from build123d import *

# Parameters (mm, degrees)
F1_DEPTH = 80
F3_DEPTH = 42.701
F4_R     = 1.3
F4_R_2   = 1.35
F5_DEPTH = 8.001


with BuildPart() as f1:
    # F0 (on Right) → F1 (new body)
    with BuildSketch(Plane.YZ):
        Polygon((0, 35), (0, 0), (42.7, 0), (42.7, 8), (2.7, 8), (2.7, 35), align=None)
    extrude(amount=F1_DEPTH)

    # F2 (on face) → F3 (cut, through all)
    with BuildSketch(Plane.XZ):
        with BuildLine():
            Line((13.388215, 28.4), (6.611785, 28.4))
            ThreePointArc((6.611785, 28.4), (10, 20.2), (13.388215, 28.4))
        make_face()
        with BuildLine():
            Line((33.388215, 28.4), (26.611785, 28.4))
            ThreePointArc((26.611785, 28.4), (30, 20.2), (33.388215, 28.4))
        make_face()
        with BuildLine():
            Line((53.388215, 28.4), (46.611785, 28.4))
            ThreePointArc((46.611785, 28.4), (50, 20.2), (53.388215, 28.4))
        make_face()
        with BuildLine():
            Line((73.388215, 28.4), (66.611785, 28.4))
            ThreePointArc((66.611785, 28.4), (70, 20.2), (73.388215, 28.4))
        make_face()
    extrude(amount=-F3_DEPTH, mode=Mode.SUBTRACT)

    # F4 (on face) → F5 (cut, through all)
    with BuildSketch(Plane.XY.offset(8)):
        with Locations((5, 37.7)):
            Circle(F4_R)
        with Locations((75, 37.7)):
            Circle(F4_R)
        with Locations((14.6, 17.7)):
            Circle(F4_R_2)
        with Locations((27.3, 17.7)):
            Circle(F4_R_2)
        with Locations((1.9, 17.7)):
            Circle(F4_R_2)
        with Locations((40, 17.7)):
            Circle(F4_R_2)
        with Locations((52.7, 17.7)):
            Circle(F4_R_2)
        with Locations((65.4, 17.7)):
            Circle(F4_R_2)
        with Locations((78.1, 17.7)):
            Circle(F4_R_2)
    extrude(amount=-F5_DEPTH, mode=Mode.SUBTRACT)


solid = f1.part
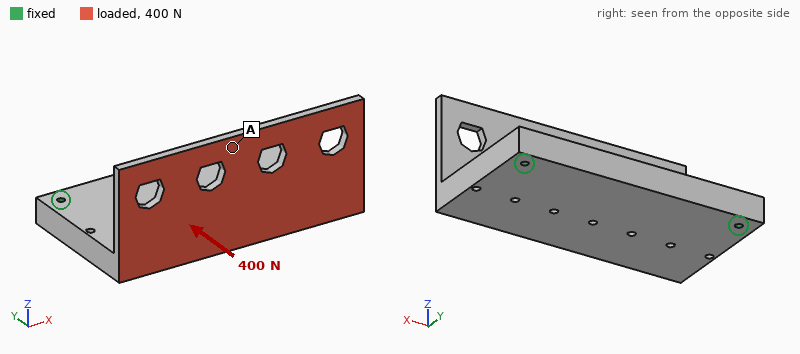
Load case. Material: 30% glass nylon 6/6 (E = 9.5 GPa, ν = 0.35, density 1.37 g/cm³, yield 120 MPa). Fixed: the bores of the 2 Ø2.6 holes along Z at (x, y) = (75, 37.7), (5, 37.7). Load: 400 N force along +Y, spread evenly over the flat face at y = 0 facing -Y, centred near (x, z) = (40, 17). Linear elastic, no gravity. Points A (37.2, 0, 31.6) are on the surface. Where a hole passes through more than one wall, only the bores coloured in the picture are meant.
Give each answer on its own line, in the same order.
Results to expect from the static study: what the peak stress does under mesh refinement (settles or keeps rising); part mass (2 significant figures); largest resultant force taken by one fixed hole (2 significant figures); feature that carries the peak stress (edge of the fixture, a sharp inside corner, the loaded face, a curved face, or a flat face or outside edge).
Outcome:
keeps rising
44 g
220 N
edge of the fixture
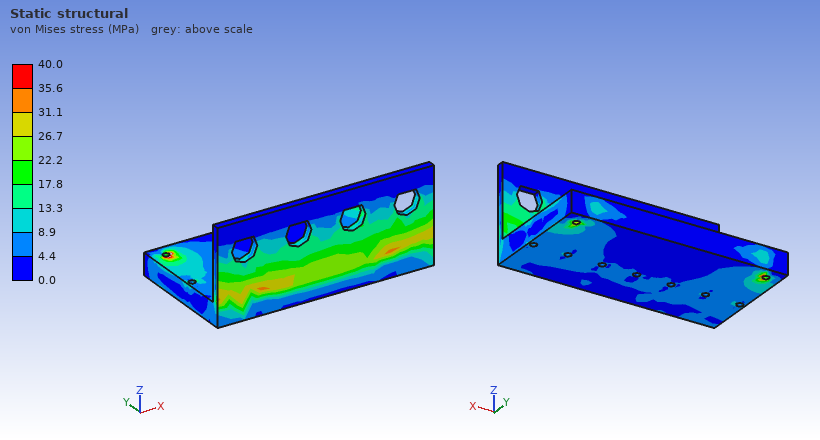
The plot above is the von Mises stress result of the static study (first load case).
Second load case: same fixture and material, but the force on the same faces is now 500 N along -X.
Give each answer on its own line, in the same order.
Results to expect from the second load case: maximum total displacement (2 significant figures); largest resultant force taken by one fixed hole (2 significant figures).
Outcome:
0.17 mm
380 N
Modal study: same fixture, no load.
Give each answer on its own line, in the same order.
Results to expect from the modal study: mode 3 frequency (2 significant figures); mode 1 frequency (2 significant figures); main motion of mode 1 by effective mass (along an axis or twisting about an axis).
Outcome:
1700 Hz
950 Hz
along Z
